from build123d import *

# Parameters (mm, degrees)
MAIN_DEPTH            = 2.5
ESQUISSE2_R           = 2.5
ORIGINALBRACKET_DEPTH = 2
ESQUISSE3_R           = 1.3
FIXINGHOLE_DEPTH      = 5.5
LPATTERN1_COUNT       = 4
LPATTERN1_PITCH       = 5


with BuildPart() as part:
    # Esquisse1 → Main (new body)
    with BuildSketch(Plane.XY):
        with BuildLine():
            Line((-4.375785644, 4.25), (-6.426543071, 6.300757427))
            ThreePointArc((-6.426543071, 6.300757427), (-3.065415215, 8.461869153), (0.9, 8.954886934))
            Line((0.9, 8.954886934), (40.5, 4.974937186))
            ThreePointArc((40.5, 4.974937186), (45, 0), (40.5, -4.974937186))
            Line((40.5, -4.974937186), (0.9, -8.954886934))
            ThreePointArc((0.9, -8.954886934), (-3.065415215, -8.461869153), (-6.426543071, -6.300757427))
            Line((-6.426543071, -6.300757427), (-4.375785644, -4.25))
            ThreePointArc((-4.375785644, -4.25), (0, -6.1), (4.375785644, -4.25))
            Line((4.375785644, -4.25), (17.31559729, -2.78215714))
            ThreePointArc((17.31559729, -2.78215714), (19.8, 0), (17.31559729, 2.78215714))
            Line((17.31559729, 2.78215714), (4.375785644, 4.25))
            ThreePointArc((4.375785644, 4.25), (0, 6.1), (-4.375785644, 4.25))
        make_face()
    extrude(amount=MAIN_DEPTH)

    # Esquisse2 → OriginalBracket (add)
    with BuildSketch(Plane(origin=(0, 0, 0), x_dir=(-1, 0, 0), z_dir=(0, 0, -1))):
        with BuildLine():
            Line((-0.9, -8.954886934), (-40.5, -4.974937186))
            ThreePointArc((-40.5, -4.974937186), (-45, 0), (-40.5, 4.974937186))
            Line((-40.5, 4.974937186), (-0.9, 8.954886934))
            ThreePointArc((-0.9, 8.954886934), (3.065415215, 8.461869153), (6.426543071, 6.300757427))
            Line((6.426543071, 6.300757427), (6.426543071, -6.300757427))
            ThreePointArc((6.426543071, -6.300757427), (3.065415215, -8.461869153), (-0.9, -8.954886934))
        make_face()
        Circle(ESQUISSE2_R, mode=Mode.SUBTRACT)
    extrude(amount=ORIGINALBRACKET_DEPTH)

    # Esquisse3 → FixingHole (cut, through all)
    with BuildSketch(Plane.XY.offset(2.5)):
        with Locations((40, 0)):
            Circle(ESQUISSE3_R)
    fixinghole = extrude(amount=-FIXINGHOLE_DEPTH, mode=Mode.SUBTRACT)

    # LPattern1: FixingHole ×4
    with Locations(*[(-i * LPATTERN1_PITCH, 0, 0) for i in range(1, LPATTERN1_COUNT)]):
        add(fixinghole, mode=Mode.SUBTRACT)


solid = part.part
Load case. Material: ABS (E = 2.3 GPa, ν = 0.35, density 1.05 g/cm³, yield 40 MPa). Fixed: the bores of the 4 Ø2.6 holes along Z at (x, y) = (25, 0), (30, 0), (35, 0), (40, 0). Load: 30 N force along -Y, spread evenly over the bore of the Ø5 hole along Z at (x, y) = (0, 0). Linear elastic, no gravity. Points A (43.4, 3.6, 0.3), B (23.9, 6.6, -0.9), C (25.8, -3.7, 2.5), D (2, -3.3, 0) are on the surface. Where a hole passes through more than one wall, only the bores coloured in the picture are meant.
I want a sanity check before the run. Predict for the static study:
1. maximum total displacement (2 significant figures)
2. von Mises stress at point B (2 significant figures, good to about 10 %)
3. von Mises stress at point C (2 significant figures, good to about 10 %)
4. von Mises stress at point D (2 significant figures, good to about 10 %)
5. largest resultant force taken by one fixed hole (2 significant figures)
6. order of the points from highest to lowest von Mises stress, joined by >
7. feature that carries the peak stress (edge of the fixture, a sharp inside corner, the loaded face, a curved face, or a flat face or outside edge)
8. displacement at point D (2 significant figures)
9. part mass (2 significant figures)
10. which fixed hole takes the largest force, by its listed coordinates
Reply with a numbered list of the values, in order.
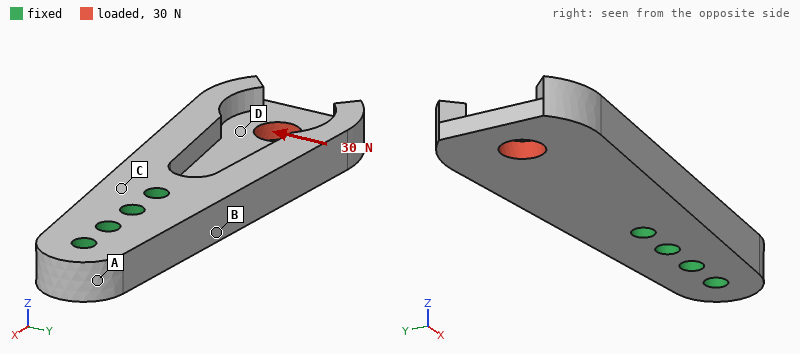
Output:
1. 0.22 mm
2. 5.8 MPa
3. 3.5 MPa
4. 1.9 MPa
5. 91 N
6. B > C > D > A
7. edge of the fixture
8. 0.15 mm
9. 2.6 g
10. (25, 0)
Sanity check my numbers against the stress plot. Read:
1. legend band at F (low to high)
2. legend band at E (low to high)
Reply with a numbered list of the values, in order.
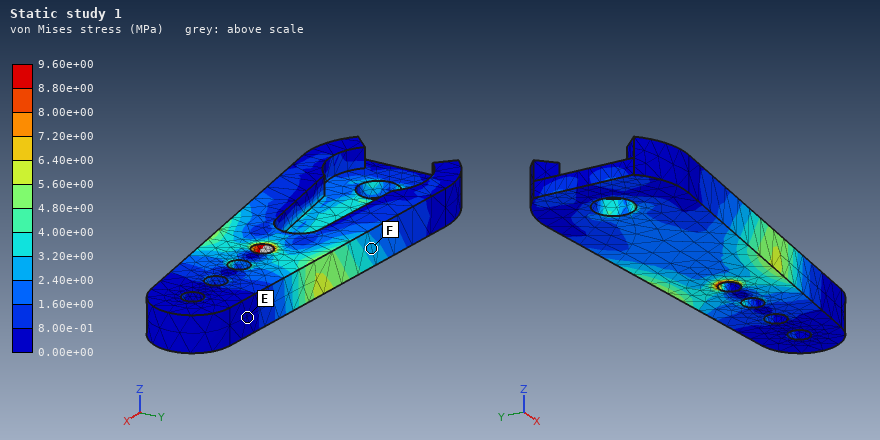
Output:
1. 2.40e+00 to 3.20e+00 MPa
2. 0.00e+00 to 8.00e-01 MPa
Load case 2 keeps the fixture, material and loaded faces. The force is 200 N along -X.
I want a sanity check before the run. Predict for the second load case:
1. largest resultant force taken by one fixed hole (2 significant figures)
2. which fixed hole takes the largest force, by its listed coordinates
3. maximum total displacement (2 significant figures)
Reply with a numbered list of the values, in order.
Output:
1. 140 N
2. (25, 0)
3. 0.46 mm
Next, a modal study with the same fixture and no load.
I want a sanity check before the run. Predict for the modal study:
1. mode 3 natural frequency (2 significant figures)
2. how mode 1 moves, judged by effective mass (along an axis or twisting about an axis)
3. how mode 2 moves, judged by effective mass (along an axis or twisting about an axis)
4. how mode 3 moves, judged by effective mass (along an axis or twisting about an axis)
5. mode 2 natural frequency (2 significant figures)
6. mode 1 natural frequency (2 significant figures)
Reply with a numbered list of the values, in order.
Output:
1. 2700 Hz
2. along Z
3. along Y
4. along Y
5. 2200 Hz
6. 1100 Hz
